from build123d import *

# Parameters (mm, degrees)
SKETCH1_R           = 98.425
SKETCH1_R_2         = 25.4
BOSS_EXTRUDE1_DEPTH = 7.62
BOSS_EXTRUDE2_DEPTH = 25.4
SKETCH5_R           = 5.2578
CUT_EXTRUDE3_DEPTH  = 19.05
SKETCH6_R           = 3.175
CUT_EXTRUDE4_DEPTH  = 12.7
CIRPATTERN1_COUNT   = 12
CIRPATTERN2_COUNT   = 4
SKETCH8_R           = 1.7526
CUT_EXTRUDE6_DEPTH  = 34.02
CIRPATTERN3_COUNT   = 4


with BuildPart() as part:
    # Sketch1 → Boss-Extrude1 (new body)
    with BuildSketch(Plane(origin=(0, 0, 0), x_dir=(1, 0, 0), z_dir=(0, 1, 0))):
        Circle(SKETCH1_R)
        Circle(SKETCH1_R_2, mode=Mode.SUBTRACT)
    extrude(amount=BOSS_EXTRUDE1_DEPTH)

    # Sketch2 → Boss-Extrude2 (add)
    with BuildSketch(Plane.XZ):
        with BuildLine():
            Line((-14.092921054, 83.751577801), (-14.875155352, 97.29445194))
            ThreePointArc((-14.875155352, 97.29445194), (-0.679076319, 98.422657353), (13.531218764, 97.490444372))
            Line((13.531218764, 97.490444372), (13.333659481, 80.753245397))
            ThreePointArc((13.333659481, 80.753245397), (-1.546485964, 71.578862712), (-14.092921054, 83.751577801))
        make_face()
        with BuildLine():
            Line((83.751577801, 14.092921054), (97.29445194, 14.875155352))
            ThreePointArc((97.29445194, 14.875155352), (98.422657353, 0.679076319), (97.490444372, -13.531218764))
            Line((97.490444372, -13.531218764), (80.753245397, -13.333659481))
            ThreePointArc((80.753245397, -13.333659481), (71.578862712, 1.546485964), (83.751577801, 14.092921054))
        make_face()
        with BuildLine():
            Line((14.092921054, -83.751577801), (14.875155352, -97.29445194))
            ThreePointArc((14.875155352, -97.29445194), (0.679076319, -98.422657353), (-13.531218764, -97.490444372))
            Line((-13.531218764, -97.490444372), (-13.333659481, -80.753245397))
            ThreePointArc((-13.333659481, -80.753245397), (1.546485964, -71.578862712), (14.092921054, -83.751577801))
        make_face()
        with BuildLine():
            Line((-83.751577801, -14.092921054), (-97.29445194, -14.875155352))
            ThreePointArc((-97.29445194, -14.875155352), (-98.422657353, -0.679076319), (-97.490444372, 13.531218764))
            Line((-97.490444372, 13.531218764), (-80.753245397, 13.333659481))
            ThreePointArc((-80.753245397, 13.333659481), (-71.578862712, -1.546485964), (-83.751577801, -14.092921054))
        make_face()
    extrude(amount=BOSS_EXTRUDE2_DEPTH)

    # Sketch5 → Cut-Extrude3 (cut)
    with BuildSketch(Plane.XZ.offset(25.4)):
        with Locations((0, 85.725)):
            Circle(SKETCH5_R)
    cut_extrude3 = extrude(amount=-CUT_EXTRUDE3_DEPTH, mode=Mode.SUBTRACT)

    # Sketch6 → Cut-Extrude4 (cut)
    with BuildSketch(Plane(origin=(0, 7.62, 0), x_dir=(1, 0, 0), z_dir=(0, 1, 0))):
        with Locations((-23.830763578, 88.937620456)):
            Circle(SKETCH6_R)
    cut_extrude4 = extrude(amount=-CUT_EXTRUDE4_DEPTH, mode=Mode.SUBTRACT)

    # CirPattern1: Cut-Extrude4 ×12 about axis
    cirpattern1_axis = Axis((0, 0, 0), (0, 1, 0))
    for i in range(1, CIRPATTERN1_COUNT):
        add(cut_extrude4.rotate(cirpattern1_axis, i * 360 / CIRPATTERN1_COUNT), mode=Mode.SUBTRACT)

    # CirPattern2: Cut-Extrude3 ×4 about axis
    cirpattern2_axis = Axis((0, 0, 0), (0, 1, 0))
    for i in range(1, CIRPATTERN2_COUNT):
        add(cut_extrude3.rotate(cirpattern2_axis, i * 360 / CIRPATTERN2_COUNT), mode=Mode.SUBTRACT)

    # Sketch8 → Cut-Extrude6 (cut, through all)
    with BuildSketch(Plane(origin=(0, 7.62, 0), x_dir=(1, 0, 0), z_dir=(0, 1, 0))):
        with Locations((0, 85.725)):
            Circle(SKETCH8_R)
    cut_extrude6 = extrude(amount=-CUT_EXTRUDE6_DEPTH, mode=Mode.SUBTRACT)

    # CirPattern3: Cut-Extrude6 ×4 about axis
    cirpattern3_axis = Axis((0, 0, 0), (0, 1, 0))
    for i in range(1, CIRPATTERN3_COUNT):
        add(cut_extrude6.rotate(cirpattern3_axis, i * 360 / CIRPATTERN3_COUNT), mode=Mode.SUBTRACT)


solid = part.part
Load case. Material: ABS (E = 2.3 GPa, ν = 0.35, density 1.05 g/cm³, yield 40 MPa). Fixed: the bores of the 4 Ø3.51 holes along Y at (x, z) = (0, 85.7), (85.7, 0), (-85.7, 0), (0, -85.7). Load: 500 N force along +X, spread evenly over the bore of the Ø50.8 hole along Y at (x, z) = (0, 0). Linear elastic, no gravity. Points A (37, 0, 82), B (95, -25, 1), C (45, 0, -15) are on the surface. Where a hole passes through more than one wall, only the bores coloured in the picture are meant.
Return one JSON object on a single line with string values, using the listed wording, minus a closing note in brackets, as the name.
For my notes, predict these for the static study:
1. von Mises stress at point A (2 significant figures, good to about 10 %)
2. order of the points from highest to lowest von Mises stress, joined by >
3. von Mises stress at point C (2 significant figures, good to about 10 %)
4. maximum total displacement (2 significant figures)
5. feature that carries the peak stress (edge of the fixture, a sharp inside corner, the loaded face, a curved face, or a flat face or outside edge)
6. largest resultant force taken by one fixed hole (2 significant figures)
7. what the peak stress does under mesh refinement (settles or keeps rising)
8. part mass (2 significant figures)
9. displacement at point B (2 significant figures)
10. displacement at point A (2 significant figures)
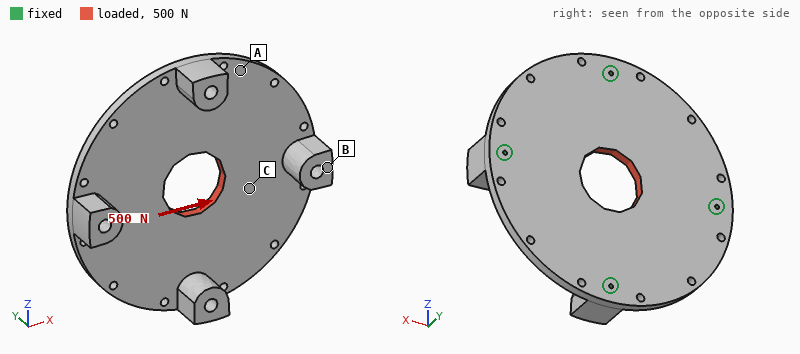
{"von Mises stress at point A": "0.18 MPa", "order of the points from highest to lowest von Mises stress, joined by >": "C > A > B", "von Mises stress at point C": "0.46 MPa", "maximum total displacement": "18 µm", "feature that carries the peak stress": "edge of the fixture", "largest resultant force taken by one fixed hole": "160 N", "what the peak stress does under mesh refinement": "keeps rising", "part mass": "290 g", "displacement at point B": "3.9 µm", "displacement at point A": "6.6 µm"}
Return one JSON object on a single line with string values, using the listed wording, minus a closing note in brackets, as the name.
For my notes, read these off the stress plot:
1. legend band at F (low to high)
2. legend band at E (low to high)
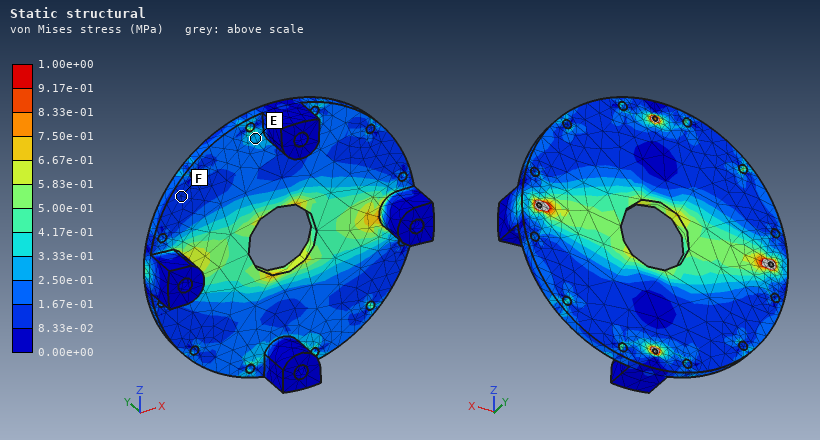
{"legend band at F": "8.33e-02 to 1.67e-01 MPa", "legend band at E": "2.50e-01 to 3.33e-01 MPa"}
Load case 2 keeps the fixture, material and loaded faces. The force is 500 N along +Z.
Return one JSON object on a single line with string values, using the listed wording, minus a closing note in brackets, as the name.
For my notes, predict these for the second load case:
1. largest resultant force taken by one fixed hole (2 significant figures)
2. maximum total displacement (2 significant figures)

{"largest resultant force taken by one fixed hole": "160 N", "maximum total displacement": "18 µm"}
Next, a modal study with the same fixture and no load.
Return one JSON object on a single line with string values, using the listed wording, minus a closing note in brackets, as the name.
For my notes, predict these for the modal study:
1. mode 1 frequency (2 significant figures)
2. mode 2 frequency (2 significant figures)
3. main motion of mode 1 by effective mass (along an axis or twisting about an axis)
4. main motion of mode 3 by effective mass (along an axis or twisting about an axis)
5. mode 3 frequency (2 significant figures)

{"mode 1 frequency": "680 Hz", "mode 2 frequency": "710 Hz", "main motion of mode 1 by effective mass": "along Y", "main motion of mode 3 by effective mass": "twisting about X", "mode 3 frequency": "770 Hz"}
